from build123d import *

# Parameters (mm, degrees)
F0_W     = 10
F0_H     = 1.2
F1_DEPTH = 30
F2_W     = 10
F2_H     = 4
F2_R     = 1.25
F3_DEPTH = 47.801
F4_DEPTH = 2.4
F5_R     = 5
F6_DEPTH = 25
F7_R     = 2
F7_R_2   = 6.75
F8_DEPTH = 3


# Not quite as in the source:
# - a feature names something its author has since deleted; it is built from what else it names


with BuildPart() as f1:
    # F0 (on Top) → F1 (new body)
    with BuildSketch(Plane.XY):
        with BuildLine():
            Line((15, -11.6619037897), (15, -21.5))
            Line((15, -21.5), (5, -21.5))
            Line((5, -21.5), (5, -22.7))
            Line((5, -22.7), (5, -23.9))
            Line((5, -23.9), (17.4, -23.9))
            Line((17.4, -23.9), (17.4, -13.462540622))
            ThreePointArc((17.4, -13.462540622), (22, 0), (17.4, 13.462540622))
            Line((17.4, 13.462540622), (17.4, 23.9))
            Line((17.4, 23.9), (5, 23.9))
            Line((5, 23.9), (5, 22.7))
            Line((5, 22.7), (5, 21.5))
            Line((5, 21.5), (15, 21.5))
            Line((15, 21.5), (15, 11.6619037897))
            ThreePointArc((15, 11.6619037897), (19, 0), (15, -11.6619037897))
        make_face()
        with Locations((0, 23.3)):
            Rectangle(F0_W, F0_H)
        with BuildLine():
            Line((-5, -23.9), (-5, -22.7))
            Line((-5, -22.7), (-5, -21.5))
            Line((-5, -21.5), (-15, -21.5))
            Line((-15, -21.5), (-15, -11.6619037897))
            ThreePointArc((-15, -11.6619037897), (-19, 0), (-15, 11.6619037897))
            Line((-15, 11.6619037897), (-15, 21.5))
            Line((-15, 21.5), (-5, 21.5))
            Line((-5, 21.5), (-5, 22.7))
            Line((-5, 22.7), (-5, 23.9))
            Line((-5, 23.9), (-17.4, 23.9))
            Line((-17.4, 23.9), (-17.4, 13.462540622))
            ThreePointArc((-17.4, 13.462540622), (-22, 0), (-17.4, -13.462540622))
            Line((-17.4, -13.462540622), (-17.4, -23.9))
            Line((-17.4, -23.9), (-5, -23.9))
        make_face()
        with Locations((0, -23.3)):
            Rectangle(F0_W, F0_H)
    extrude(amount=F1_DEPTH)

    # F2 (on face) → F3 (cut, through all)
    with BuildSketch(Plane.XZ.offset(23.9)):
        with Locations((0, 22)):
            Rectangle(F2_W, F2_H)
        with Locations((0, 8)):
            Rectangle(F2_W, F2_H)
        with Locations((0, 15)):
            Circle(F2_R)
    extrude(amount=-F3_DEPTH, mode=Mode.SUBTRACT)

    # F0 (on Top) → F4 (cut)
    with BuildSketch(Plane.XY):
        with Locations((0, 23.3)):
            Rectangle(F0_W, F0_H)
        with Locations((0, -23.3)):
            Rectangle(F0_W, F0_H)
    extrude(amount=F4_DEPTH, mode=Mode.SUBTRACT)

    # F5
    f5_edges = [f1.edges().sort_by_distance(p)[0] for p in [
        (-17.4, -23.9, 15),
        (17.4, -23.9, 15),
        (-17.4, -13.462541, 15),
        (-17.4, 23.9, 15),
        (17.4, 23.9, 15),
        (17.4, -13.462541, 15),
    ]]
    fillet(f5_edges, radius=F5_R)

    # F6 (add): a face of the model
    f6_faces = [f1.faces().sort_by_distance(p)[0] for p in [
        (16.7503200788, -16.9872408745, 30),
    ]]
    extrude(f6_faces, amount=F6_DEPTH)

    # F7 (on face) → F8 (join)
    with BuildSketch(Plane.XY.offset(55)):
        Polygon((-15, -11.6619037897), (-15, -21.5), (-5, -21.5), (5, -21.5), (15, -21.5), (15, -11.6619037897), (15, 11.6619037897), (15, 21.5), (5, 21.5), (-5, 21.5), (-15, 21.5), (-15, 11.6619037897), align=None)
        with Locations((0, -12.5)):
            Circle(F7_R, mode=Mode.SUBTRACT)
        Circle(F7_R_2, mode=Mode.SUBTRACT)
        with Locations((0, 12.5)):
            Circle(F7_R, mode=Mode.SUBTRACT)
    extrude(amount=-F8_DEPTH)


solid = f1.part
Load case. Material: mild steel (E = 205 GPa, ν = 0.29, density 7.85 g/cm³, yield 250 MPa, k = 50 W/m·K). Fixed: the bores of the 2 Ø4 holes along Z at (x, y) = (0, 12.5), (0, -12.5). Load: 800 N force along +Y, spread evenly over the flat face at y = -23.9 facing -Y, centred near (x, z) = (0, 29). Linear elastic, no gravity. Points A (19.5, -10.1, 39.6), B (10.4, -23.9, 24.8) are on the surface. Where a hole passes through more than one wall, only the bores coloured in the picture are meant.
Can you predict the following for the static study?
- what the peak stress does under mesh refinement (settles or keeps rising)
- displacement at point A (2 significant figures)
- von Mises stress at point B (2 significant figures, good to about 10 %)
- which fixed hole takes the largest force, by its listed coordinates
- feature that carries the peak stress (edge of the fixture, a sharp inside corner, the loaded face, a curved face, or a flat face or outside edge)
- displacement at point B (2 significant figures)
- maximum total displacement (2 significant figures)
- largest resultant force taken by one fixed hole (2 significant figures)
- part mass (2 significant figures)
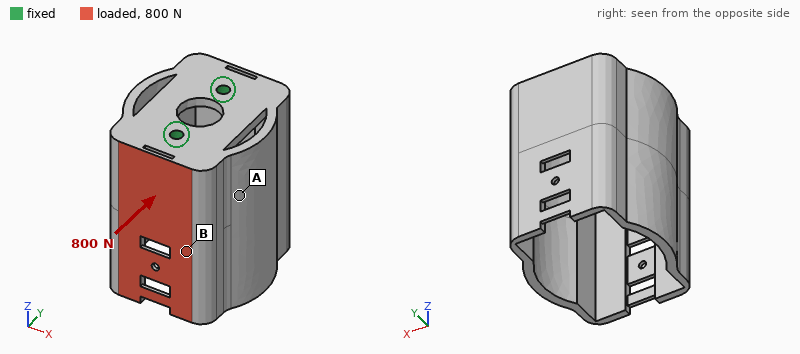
keeps rising
13 µm
17 MPa
(0, -12.5)
edge of the fixture
38 µm
82 µm
750 N
180 g
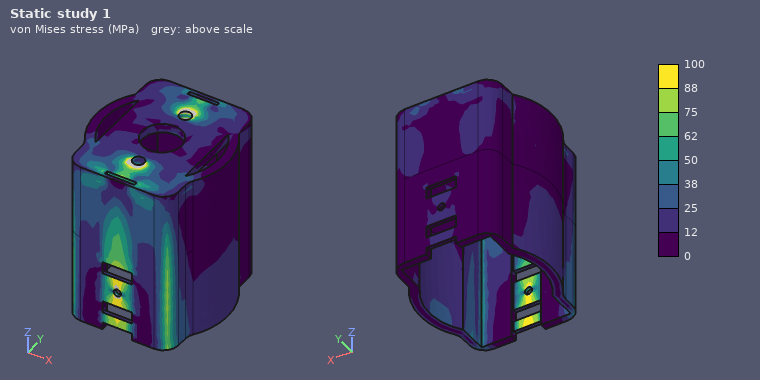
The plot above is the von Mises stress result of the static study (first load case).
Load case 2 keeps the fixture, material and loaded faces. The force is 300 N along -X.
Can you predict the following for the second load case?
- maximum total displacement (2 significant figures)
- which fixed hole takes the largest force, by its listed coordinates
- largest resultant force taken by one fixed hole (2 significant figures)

78 µm
(0, -12.5)
390 N
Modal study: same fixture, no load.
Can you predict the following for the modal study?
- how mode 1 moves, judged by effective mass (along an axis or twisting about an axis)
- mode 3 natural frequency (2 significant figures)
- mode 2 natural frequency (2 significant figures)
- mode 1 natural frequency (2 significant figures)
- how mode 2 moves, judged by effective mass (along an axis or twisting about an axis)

along X
2300 Hz
2000 Hz
920 Hz
along Y
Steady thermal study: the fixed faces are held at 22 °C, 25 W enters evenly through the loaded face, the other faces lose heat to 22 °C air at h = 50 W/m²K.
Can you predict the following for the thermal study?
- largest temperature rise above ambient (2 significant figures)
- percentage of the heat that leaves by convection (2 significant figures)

53 K
66 %
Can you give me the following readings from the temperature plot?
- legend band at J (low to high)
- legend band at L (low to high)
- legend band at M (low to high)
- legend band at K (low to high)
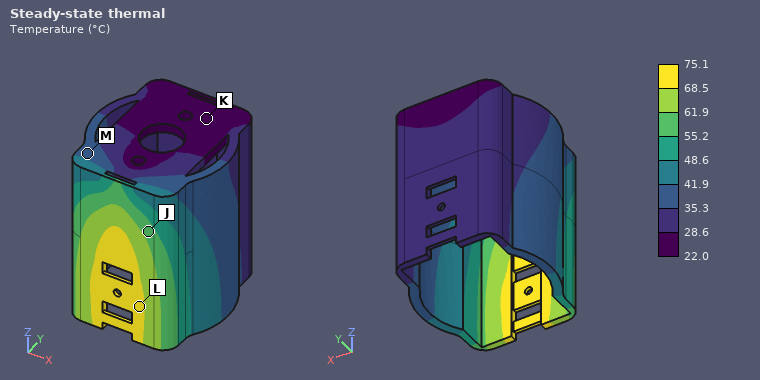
55.2 to 61.9 °C
68.5 to 75.1 °C
35.3 to 41.9 °C
22.0 to 28.6 °C
